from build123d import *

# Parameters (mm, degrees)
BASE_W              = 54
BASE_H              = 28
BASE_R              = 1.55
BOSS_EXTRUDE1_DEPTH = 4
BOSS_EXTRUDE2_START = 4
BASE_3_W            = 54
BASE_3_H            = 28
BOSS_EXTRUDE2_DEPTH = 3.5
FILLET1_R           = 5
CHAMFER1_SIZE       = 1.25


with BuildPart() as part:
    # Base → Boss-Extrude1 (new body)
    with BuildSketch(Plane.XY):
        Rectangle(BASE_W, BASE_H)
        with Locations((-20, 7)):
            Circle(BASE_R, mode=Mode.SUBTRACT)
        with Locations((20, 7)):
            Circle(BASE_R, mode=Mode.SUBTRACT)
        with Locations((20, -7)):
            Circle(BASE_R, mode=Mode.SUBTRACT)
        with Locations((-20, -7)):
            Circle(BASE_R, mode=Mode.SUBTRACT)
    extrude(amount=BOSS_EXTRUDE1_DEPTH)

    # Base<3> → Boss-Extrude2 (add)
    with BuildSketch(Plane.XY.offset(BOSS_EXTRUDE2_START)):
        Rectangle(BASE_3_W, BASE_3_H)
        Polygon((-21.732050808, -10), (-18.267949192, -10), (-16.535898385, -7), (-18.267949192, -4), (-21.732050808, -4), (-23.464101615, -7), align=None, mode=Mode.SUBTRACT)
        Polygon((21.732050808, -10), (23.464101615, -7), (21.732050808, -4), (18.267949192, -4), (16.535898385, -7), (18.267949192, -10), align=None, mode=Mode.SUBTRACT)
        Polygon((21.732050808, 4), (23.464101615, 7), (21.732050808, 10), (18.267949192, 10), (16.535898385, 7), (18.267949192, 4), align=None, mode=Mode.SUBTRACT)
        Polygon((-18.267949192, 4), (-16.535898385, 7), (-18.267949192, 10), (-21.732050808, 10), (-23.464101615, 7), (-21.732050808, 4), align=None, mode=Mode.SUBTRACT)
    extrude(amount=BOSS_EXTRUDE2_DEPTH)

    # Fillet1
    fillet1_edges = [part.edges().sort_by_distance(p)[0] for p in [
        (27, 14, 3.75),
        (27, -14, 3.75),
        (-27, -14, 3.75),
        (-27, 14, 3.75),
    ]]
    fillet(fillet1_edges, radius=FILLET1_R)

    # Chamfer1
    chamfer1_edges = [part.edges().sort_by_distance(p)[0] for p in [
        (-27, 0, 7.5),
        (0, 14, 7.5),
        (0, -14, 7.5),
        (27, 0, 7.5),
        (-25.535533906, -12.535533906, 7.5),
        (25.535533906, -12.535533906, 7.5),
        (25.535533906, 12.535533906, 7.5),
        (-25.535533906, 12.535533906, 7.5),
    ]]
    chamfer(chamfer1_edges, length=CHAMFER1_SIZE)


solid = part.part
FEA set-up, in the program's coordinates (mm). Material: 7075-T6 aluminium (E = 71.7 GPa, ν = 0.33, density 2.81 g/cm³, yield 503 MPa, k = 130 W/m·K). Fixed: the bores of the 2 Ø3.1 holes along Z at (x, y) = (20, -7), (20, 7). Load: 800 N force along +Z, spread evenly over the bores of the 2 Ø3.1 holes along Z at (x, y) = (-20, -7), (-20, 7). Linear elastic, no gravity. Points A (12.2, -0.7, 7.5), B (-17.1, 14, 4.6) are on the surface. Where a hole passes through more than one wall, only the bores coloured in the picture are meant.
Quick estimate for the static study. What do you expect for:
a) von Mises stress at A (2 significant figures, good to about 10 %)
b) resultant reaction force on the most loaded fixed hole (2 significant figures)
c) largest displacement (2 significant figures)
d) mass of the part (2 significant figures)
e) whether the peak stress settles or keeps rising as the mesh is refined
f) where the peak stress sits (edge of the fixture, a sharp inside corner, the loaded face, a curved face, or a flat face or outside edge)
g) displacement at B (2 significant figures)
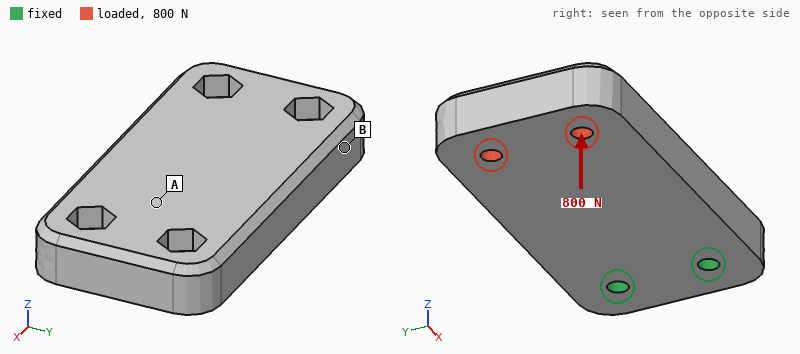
110 MPa
490 N
0.55 mm
30 g
keeps rising
edge of the fixture
0.40 mm
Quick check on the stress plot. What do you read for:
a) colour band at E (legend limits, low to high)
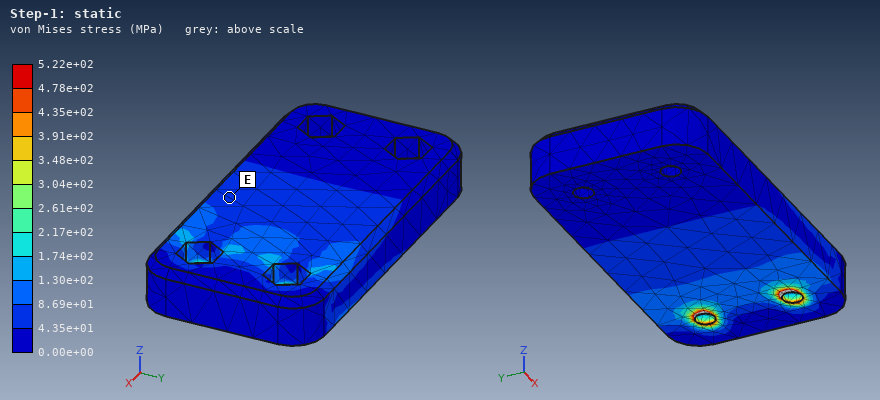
4.35e+01 to 8.69e+01 MPa
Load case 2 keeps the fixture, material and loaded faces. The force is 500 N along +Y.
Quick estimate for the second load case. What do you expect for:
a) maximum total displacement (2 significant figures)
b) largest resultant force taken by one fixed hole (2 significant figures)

34 µm
1.3 kN
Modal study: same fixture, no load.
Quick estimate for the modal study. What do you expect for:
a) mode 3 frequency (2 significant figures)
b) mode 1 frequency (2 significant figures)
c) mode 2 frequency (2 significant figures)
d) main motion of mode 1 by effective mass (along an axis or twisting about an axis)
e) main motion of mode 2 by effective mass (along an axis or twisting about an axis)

8400 Hz
2100 Hz
6600 Hz
along Z
along Y
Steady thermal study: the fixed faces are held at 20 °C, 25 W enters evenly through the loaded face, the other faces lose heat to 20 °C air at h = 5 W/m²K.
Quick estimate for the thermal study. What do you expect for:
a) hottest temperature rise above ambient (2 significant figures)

45 K
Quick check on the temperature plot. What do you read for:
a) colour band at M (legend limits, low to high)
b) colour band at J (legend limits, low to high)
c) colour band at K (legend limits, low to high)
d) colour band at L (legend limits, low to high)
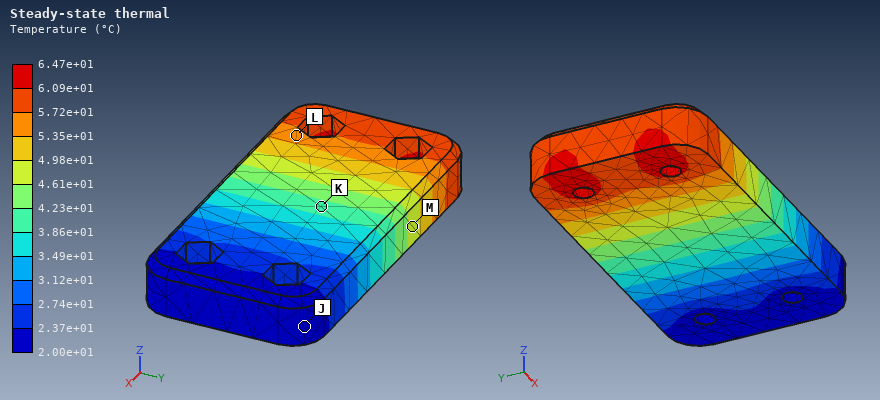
4.61e+01 to 4.98e+01 °C
2.00e+01 to 2.37e+01 °C
3.86e+01 to 4.23e+01 °C
5.35e+01 to 5.72e+01 °C
